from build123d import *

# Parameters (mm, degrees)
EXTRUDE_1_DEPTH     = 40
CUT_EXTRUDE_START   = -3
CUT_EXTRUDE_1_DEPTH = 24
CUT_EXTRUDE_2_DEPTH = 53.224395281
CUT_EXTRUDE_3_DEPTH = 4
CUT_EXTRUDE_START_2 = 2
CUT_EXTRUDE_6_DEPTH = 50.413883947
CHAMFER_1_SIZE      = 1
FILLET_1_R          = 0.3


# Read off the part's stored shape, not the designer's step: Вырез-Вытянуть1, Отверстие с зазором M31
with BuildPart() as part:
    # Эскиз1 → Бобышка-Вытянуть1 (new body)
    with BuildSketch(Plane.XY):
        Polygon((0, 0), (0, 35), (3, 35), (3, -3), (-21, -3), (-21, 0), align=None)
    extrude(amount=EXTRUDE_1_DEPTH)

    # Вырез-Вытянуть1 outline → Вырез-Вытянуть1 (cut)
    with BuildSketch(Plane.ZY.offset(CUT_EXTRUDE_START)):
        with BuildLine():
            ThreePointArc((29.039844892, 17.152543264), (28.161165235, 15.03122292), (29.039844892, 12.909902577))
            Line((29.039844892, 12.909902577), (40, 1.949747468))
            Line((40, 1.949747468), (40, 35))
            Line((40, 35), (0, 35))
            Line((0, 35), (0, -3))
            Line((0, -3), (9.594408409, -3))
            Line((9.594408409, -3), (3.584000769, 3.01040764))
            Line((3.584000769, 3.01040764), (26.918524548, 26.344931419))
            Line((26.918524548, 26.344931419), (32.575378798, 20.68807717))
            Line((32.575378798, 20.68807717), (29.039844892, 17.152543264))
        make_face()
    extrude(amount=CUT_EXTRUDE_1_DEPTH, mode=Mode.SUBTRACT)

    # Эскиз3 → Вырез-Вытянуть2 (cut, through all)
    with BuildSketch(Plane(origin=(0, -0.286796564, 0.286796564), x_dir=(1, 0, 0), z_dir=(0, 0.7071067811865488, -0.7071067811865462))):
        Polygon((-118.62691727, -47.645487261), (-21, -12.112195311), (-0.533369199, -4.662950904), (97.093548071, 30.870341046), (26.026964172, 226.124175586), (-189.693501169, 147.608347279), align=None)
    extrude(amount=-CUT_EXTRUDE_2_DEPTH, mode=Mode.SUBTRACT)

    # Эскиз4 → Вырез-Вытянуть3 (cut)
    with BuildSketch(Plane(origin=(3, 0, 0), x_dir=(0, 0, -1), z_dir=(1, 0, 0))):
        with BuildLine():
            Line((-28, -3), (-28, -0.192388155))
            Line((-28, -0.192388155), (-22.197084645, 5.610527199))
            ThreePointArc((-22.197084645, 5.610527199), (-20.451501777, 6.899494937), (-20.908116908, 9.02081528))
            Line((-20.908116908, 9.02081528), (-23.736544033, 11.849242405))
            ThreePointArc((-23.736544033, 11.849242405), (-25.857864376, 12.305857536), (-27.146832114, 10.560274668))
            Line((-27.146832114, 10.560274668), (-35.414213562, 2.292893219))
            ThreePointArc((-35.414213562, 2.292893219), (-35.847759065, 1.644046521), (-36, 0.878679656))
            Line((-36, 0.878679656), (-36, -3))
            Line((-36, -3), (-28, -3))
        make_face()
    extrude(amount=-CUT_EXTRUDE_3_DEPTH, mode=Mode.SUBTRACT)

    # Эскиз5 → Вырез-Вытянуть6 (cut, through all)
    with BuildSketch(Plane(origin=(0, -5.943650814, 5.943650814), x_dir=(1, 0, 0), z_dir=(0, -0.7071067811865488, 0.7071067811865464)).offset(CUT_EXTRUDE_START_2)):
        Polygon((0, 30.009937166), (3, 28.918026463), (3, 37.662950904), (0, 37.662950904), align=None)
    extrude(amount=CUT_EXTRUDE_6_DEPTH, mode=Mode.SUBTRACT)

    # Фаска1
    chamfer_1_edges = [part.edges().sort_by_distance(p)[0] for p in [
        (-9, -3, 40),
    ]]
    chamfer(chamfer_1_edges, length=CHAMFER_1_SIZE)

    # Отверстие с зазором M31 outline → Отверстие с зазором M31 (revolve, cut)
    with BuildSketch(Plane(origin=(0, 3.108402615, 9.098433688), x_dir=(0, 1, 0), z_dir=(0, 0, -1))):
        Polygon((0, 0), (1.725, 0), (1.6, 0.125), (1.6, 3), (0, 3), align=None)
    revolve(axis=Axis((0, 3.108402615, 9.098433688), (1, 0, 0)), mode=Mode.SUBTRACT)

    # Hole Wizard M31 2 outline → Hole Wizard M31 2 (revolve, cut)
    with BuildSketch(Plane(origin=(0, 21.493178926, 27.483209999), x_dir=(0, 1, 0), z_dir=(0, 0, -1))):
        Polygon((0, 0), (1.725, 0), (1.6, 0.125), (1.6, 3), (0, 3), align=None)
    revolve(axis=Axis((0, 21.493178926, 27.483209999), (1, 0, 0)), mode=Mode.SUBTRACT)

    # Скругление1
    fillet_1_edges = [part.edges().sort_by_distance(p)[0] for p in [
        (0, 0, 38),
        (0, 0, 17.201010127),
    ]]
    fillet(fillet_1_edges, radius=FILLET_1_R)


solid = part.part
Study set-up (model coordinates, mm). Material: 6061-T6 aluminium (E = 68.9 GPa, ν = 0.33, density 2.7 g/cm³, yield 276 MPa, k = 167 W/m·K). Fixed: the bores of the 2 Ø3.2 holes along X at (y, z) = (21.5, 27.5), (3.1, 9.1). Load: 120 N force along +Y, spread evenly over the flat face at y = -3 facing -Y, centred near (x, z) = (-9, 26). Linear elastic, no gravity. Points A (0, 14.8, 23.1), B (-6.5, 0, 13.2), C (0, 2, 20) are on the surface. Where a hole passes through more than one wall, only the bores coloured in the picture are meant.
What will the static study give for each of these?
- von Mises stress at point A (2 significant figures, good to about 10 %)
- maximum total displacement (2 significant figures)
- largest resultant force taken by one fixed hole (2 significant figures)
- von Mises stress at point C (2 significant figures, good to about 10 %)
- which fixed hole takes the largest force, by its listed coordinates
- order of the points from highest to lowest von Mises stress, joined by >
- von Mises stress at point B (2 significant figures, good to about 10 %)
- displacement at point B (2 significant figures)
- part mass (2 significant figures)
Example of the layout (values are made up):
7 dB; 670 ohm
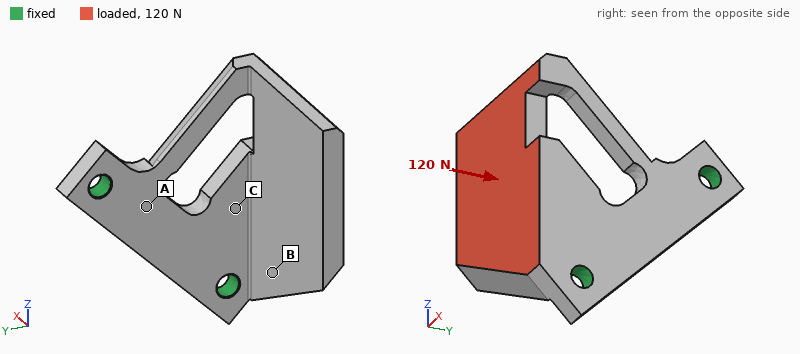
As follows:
6.6 MPa; 0.15 mm; 86 N; 38 MPa; (21.5, 27.5); C > B > A; 23 MPa; 0.027 mm; 8.0 g
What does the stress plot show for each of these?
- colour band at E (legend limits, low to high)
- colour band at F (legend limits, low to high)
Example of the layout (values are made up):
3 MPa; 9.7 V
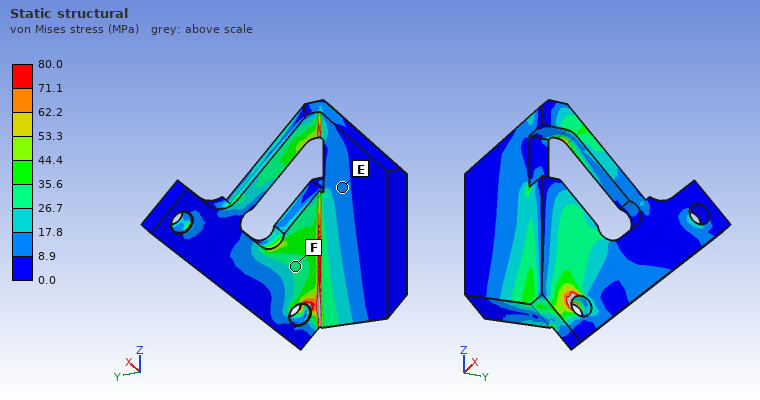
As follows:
8.9 to 17.8 MPa; 26.7 to 35.6 MPa
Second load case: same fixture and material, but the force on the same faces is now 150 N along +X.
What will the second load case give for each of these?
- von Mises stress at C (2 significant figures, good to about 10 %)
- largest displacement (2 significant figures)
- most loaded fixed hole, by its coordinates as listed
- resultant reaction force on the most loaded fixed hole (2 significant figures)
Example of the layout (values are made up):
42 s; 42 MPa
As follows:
18 MPa; 0.17 mm; (3.1, 9.1); 130 N
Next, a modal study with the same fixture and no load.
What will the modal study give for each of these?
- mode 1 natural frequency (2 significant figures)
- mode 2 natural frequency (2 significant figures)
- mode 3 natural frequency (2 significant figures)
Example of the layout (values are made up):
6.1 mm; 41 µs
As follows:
2300 Hz; 3400 Hz; 9600 Hz
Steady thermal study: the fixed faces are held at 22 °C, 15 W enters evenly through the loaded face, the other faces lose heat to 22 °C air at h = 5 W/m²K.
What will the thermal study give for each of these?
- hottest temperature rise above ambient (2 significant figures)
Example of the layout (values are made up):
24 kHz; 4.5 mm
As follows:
33 K
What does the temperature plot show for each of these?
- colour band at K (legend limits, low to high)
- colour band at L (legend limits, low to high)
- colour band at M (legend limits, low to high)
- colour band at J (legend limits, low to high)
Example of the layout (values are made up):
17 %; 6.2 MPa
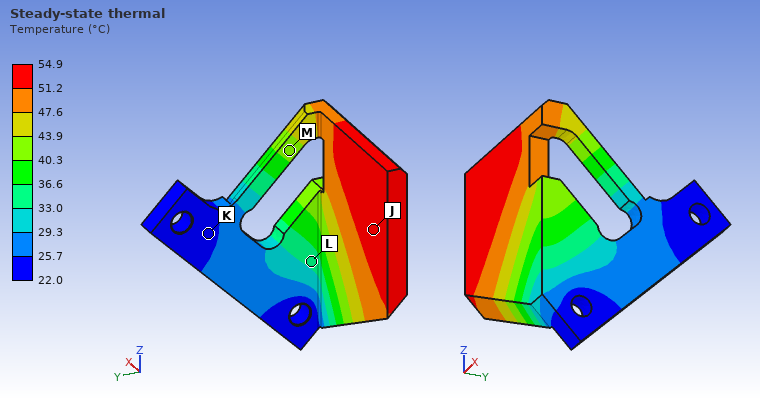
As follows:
22.0 to 25.7 °C; 33.0 to 36.6 °C; 40.3 to 43.9 °C; 51.2 to 54.9 °C
